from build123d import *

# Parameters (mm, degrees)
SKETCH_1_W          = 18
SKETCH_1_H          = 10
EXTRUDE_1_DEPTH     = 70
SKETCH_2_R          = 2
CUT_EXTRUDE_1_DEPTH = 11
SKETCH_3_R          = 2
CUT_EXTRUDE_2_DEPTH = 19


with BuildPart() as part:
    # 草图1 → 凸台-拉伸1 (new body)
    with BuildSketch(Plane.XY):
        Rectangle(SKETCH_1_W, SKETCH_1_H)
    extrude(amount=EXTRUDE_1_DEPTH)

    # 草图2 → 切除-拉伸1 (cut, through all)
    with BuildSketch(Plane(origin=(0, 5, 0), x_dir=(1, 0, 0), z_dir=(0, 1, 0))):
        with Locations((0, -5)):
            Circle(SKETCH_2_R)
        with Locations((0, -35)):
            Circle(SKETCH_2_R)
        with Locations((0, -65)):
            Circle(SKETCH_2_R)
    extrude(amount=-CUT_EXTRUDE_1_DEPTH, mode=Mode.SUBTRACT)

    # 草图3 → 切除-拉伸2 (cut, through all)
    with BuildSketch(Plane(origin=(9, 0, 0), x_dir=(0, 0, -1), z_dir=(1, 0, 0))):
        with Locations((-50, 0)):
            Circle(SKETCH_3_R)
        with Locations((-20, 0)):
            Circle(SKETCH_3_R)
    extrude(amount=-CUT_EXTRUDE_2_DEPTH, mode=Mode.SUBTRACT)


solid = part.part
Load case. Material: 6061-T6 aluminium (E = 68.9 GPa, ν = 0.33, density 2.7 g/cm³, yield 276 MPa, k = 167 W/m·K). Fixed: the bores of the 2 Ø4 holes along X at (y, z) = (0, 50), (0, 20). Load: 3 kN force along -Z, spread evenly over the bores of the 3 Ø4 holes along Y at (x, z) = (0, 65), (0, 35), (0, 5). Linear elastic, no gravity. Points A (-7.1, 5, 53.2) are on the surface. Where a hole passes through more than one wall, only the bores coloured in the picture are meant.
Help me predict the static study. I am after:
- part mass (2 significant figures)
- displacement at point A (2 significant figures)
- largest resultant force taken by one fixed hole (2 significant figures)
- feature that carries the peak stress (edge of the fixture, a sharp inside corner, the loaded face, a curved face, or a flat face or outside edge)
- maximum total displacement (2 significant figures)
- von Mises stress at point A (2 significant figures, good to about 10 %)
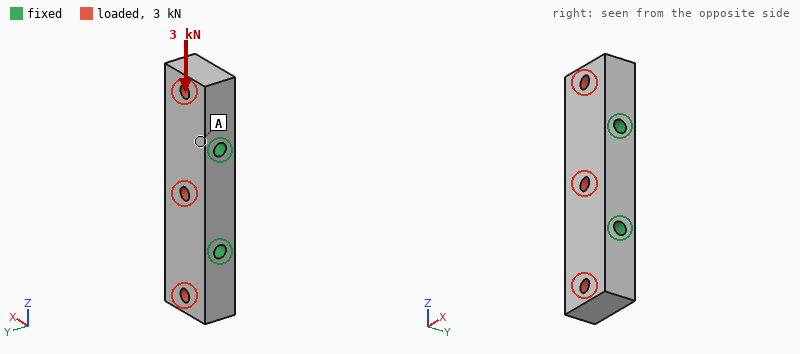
32 g
0.42 µm
1.5 kN
the loaded face
2.3 µm
2.4 MPa
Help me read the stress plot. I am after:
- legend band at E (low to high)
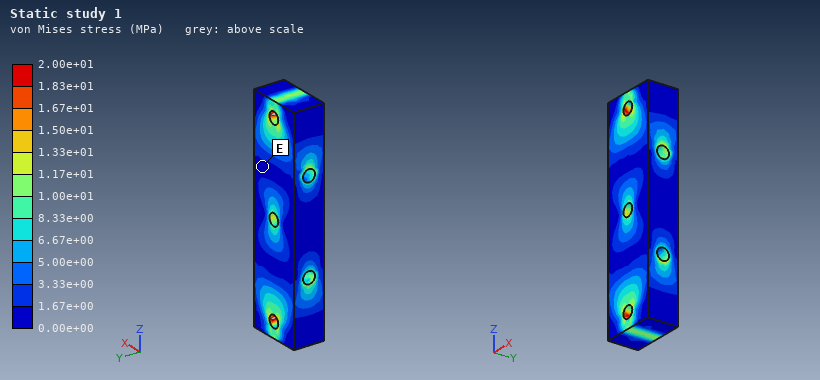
0.00e+00 to 1.67e+00 MPa
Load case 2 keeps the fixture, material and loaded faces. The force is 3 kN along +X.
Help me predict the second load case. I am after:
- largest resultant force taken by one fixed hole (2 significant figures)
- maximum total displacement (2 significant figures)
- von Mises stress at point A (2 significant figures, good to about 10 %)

1.5 kN
9.3 µm
11 MPa
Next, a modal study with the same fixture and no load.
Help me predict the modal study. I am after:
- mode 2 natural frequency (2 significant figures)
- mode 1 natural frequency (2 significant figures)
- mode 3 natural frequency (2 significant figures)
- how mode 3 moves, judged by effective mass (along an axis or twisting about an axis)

16 kHz
16 kHz
26 kHz
along X
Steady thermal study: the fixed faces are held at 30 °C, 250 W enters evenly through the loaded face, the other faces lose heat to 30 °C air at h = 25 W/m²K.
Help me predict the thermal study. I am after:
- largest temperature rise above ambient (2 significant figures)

49 K
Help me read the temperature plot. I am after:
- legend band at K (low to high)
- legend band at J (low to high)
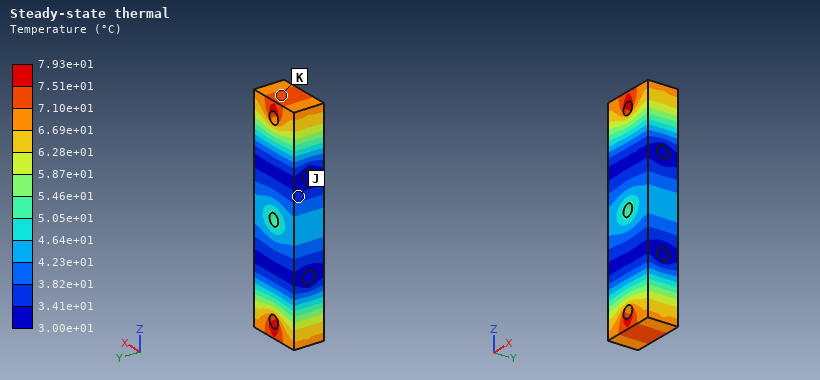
7.10e+01 to 7.51e+01 °C
3.41e+01 to 3.82e+01 °C
